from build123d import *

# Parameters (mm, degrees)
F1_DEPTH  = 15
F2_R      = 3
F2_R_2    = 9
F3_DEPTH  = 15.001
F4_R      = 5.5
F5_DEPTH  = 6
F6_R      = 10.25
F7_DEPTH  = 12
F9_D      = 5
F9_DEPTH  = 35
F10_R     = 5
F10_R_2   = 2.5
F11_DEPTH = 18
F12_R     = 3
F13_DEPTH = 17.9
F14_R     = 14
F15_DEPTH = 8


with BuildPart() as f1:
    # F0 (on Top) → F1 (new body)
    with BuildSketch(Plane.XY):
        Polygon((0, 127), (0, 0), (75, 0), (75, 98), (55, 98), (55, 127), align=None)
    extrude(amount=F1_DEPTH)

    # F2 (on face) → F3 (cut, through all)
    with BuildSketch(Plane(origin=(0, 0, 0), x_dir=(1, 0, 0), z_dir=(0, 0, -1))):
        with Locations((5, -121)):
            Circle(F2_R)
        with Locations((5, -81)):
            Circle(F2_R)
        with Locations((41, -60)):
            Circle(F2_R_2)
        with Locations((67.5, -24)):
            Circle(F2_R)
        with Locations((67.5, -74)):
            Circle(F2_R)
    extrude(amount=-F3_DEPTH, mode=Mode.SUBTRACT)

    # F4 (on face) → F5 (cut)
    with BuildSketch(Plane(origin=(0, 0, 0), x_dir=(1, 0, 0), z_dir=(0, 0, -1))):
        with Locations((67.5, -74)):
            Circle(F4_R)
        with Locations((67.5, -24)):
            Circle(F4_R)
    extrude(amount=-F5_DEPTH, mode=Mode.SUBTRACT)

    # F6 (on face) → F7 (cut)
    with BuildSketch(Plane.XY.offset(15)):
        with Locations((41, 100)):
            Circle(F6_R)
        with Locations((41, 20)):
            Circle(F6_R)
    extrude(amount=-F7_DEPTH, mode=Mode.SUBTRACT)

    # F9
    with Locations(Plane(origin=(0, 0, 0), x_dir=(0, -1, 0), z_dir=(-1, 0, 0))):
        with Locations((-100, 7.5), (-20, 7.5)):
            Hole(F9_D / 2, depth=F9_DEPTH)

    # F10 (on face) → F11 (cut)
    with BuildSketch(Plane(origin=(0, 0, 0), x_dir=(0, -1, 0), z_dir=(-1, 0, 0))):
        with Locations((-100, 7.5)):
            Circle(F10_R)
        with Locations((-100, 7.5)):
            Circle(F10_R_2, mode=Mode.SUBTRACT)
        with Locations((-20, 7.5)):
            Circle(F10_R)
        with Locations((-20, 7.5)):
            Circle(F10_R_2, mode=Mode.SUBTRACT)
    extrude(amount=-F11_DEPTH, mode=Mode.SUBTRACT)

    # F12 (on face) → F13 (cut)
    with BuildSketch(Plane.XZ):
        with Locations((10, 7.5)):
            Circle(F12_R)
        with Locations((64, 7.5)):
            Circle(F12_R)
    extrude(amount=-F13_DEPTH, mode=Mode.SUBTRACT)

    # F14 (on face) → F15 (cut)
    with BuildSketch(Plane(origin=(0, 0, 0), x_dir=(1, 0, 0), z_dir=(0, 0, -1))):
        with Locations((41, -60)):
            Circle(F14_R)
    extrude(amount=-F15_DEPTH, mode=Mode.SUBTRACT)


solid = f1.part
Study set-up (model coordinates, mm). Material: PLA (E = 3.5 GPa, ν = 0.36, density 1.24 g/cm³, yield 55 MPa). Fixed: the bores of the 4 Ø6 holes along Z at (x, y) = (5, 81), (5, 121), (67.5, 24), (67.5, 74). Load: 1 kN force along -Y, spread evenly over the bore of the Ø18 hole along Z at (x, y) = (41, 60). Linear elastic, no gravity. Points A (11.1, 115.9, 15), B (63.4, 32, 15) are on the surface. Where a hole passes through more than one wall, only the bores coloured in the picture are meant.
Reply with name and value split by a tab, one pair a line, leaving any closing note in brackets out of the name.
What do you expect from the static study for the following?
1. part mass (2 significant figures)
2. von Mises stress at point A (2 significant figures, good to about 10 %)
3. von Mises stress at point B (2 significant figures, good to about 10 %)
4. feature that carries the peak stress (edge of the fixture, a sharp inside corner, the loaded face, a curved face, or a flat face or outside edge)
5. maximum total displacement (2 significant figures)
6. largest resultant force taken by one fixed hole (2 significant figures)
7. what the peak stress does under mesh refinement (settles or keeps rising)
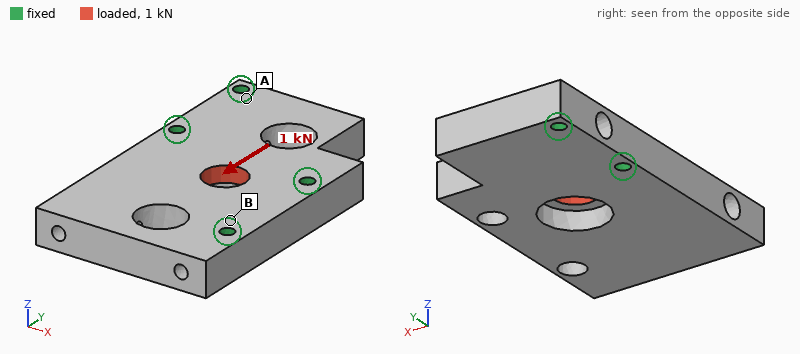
part mass	140 g
von Mises stress at point A	0.57 MPa
von Mises stress at point B	1.4 MPa
feature that carries the peak stress	edge of the fixture
maximum total displacement	34 µm
largest resultant force taken by one fixed hole	350 N
what the peak stress does under mesh refinement	keeps rising
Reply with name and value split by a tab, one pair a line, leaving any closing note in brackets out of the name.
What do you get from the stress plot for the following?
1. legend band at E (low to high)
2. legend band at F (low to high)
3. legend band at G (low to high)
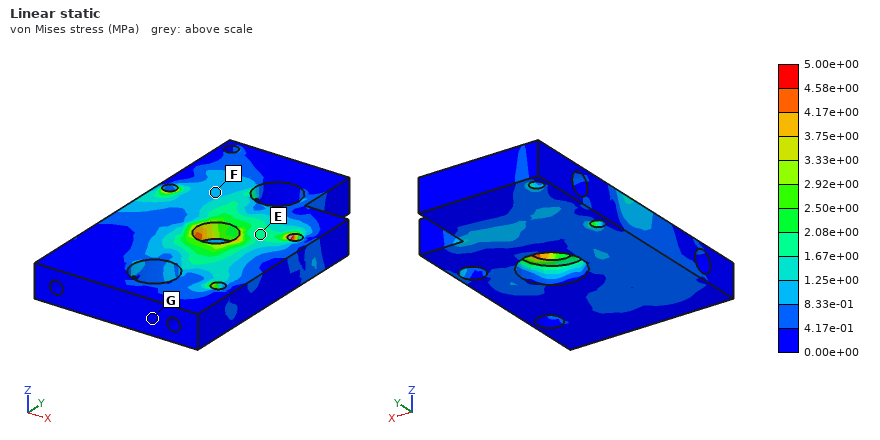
legend band at E	1.67e+00 to 2.08e+00 MPa
legend band at F	8.33e-01 to 1.25e+00 MPa
legend band at G	0.00e+00 to 4.17e-01 MPa
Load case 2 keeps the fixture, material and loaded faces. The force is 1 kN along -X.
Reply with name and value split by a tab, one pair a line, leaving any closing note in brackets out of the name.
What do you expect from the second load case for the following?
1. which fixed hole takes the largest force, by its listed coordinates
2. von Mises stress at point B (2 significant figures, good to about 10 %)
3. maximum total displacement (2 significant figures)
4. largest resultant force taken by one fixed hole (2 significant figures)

which fixed hole takes the largest force, by its listed coordinates	(67.5, 74)
von Mises stress at point B	1.6 MPa
maximum total displacement	26 µm
largest resultant force taken by one fixed hole	410 N
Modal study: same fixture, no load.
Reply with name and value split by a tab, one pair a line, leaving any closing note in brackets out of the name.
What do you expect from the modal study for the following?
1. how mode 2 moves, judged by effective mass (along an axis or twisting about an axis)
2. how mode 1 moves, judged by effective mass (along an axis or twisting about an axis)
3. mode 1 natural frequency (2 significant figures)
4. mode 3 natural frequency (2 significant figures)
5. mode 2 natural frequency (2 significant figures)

how mode 2 moves, judged by effective mass	along Z
how mode 1 moves, judged by effective mass	along Z
mode 1 natural frequency	1100 Hz
mode 3 natural frequency	3000 Hz
mode 2 natural frequency	2400 Hz
